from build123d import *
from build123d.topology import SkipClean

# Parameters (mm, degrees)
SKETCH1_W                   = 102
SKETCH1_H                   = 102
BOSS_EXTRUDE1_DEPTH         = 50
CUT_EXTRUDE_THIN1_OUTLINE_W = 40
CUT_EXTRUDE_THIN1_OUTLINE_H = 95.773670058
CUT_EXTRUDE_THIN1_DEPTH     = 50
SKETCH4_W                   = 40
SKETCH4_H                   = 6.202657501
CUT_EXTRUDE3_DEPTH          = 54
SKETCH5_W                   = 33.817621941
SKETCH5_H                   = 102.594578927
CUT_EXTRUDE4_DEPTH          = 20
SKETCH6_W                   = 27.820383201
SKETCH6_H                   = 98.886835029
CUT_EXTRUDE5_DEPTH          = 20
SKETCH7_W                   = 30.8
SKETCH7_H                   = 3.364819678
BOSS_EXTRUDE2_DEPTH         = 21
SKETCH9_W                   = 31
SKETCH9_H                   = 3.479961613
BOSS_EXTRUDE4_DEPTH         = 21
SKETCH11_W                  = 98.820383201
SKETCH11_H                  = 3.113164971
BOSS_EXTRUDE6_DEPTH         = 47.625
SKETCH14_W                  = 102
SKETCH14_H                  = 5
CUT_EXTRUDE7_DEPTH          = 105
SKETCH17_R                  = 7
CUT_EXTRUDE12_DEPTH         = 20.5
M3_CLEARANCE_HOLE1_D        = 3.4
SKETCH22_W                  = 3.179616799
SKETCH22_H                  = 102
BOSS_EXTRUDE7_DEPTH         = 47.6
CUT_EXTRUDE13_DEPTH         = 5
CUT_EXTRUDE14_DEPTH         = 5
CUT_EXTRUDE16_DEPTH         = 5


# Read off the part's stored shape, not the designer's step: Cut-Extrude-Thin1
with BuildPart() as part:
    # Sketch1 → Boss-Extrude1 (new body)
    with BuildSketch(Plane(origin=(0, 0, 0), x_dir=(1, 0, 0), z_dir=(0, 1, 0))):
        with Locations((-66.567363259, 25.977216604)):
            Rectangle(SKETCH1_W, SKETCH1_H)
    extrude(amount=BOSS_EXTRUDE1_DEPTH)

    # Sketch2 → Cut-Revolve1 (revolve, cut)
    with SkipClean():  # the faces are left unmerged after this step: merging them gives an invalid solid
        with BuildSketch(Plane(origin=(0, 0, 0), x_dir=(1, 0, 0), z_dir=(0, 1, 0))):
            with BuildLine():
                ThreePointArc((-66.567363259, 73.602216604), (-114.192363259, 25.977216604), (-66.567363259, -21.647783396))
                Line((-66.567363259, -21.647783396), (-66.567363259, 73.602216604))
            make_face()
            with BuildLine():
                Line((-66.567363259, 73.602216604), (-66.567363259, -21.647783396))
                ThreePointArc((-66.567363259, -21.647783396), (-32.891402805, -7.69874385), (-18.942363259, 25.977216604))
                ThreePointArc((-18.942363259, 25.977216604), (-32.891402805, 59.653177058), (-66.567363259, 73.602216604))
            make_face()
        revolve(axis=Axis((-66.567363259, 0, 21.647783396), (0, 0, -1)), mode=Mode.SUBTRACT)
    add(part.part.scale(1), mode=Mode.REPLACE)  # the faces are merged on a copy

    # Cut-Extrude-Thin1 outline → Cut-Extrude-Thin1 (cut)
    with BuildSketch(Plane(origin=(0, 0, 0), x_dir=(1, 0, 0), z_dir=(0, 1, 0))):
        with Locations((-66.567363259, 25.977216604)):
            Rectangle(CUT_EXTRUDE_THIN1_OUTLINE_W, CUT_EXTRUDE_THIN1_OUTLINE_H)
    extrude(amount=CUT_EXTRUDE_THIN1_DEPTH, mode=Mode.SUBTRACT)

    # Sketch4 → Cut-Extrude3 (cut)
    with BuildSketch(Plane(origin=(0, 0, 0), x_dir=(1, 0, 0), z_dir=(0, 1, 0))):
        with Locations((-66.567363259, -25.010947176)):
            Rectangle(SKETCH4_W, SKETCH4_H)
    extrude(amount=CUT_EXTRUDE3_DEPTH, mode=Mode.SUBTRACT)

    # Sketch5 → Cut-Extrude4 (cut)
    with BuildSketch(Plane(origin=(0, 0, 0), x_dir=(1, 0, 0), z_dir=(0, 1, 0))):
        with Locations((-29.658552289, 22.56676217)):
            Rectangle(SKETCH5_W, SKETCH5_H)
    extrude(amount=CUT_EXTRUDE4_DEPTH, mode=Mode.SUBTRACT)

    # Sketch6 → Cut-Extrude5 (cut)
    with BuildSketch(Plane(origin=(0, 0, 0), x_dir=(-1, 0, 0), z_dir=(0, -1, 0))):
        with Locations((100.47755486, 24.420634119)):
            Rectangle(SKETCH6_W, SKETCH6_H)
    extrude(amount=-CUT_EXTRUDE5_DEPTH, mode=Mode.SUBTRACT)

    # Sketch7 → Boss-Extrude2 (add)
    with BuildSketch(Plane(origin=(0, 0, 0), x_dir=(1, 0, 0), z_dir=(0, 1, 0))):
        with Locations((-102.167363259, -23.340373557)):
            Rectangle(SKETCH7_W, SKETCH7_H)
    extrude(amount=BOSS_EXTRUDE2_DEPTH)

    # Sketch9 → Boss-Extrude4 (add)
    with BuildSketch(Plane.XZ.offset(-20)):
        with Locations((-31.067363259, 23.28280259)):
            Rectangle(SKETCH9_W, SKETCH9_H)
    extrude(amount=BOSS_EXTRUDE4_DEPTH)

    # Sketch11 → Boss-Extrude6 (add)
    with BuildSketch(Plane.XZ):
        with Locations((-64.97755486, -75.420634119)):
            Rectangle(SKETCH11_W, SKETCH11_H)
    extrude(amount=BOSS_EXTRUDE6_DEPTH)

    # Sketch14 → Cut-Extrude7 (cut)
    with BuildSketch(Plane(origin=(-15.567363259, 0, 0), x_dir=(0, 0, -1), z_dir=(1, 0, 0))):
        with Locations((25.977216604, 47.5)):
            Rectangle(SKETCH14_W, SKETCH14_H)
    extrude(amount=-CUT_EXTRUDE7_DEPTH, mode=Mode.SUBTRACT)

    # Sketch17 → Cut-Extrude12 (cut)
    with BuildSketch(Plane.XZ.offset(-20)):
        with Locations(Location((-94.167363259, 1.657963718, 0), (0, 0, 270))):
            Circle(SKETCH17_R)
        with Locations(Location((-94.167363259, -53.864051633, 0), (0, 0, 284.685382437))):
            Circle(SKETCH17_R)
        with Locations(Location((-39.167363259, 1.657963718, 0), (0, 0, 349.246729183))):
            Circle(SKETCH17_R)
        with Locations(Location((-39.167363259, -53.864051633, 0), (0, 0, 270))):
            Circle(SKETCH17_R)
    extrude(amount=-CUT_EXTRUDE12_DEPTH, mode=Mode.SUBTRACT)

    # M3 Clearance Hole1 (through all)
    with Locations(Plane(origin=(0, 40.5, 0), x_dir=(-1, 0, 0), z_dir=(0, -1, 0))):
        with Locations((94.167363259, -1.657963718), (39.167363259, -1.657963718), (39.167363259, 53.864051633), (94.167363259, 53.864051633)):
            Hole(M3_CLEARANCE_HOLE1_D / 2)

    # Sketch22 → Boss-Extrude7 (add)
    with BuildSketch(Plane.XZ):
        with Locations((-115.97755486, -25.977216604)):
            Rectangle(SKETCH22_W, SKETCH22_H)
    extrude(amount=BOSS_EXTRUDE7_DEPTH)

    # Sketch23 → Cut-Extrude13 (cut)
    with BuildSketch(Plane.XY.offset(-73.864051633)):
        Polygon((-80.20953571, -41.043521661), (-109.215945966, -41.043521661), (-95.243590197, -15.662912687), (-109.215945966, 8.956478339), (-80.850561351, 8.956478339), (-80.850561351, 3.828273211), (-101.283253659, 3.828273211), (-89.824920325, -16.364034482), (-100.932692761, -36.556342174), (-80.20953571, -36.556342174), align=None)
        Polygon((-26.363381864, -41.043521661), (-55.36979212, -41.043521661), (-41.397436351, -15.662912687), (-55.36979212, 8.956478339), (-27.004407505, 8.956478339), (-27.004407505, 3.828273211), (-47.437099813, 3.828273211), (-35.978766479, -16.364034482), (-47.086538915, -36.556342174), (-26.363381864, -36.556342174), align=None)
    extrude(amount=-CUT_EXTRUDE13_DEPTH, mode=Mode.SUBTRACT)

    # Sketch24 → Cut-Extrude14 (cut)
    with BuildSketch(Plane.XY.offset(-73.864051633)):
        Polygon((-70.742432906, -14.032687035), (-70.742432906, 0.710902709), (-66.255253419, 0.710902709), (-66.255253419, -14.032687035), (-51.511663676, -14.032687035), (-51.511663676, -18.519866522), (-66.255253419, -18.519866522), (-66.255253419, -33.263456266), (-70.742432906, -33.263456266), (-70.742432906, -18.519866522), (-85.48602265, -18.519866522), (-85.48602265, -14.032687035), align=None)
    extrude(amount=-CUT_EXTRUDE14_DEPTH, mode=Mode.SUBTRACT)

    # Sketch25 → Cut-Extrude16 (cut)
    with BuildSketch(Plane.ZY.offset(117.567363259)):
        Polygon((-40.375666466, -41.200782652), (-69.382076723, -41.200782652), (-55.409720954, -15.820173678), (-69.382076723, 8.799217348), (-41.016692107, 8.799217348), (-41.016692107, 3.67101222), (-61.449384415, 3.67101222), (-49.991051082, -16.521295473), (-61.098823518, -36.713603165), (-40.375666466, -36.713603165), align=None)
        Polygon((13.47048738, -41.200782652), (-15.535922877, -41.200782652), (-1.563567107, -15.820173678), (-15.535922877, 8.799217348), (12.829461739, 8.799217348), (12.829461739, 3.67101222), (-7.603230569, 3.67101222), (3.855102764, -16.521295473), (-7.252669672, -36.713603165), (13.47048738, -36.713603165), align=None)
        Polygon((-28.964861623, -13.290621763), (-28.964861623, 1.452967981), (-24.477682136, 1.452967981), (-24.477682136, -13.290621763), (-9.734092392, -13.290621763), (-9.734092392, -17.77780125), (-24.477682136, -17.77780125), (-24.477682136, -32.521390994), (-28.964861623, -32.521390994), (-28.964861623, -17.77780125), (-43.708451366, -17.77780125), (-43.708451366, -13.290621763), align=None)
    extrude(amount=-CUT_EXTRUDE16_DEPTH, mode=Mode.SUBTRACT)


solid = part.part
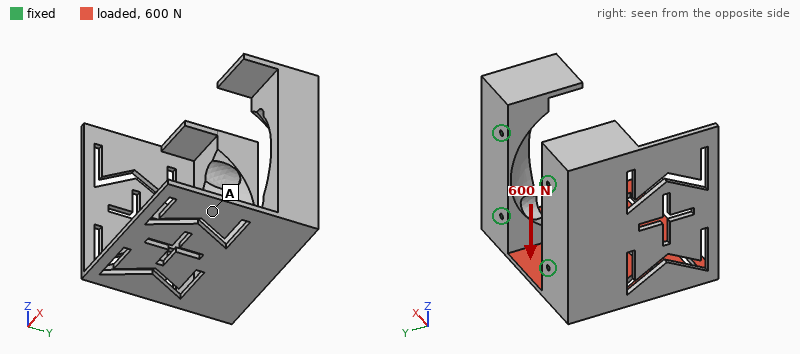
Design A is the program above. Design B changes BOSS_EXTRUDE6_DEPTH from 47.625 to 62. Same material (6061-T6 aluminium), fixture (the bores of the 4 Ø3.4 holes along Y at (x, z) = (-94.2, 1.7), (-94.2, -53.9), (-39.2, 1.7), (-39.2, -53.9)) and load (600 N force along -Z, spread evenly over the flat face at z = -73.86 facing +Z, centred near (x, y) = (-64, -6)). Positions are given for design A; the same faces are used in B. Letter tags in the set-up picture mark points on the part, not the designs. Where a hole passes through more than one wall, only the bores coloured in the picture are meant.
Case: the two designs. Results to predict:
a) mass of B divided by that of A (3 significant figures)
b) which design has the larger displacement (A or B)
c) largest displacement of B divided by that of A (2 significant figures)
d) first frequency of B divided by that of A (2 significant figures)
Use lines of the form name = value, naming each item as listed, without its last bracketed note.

mass of B divided by that of A = 1.03
which design has the larger displacement = B
largest displacement of B divided by that of A = 1.6
first frequency of B divided by that of A = 0.74
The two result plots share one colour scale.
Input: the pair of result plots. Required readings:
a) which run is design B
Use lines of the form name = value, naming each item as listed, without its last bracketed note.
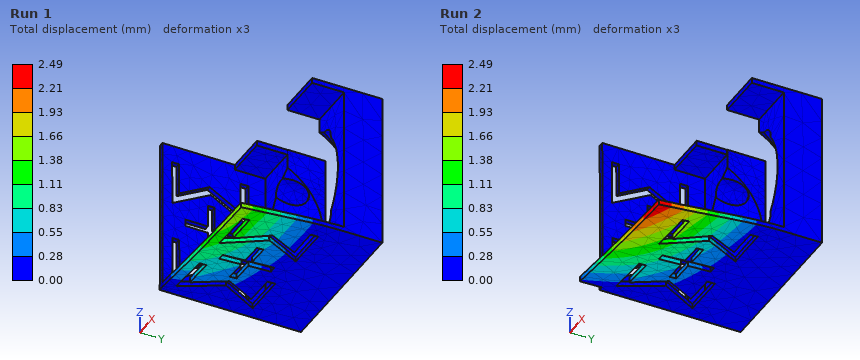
which run is design B = Run 2
